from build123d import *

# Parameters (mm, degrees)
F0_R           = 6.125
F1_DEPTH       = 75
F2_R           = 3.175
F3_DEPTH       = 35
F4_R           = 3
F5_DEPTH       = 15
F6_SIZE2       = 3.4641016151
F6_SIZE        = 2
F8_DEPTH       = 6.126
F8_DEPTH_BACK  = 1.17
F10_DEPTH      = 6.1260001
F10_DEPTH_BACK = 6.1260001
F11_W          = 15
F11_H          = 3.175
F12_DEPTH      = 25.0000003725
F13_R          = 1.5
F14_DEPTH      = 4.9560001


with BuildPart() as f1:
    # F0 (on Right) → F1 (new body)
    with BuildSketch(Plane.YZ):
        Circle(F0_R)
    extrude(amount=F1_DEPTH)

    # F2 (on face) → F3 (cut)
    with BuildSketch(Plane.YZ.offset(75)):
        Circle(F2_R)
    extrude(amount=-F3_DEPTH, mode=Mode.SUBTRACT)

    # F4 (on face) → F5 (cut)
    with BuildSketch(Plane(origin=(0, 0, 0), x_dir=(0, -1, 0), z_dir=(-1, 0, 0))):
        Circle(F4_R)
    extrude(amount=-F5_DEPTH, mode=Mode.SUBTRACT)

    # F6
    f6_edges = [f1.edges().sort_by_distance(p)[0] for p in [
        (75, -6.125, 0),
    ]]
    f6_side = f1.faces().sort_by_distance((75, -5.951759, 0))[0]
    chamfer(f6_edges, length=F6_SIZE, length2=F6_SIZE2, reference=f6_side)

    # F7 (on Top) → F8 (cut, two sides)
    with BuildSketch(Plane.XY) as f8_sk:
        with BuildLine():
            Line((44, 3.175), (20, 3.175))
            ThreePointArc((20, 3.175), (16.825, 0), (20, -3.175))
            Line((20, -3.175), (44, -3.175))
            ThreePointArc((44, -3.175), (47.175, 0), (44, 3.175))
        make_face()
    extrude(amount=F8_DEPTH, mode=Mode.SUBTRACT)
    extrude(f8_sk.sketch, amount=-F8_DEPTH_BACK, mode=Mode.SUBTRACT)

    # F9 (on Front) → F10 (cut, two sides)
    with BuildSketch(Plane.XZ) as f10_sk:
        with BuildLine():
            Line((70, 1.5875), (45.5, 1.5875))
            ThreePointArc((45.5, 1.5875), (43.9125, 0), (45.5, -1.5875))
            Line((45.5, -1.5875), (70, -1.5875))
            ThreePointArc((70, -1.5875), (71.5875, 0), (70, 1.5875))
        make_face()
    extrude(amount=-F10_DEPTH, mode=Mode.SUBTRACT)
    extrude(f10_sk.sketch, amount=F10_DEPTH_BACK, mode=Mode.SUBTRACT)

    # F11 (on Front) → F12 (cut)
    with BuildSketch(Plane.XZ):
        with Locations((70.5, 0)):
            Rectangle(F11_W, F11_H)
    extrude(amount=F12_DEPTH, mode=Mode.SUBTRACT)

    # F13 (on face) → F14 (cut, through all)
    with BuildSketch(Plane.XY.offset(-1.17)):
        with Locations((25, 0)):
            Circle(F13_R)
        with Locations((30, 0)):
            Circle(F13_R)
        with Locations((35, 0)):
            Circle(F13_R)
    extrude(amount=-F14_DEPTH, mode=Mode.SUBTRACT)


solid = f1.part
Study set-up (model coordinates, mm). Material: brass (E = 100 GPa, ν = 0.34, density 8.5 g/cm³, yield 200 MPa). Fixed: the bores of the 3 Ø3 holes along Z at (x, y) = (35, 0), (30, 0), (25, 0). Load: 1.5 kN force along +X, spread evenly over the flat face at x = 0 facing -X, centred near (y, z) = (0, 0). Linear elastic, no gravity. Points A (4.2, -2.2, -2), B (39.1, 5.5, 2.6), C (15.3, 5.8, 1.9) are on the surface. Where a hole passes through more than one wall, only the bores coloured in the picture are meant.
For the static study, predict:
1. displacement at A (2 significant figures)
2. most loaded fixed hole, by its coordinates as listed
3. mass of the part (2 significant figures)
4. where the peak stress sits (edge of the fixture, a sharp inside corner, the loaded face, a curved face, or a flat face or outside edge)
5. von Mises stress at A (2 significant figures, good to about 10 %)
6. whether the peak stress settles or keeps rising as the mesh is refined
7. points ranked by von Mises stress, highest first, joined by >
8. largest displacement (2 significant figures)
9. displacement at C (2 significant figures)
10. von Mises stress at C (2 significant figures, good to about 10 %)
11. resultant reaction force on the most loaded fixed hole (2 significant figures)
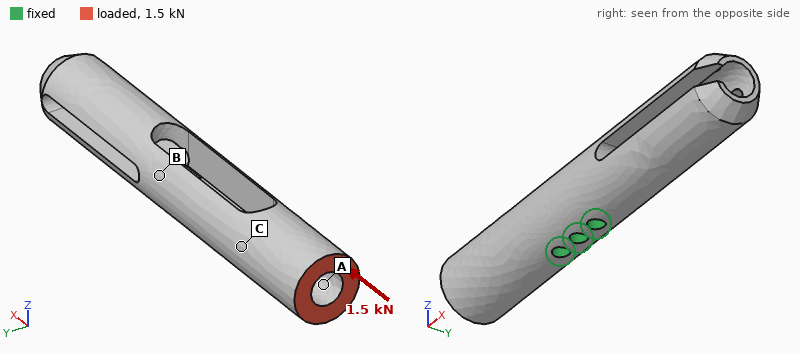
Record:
15 µm
(25, 0)
46 g
edge of the fixture
17 MPa
keeps rising
C > A > B
21 µm
7.8 µm
26 MPa
900 N
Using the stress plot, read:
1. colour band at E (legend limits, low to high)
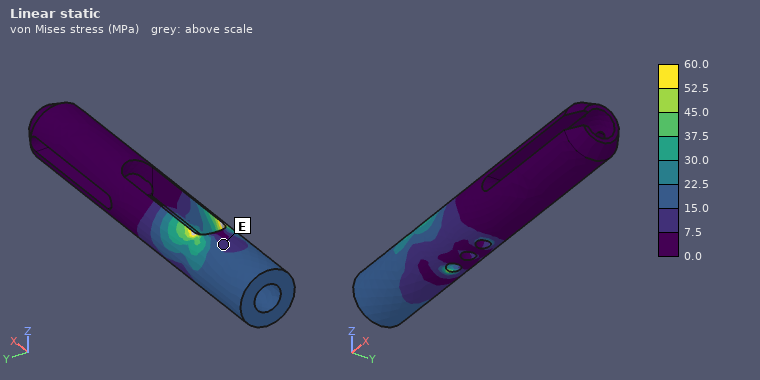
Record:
7.5 to 15.0 MPa
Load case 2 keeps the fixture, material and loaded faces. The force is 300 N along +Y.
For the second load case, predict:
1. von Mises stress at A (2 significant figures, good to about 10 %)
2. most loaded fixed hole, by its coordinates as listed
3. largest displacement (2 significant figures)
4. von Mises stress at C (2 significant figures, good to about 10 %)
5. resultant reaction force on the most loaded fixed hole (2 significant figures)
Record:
11 MPa
(25, 0)
34 µm
28 MPa
800 N
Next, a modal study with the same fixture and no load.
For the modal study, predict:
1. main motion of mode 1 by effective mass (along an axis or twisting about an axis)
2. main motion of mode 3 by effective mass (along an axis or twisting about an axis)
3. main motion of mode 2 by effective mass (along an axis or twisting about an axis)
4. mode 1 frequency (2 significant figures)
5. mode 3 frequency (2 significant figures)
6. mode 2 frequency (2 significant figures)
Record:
along Z
along Z
along Y
2000 Hz
5700 Hz
3100 Hz
